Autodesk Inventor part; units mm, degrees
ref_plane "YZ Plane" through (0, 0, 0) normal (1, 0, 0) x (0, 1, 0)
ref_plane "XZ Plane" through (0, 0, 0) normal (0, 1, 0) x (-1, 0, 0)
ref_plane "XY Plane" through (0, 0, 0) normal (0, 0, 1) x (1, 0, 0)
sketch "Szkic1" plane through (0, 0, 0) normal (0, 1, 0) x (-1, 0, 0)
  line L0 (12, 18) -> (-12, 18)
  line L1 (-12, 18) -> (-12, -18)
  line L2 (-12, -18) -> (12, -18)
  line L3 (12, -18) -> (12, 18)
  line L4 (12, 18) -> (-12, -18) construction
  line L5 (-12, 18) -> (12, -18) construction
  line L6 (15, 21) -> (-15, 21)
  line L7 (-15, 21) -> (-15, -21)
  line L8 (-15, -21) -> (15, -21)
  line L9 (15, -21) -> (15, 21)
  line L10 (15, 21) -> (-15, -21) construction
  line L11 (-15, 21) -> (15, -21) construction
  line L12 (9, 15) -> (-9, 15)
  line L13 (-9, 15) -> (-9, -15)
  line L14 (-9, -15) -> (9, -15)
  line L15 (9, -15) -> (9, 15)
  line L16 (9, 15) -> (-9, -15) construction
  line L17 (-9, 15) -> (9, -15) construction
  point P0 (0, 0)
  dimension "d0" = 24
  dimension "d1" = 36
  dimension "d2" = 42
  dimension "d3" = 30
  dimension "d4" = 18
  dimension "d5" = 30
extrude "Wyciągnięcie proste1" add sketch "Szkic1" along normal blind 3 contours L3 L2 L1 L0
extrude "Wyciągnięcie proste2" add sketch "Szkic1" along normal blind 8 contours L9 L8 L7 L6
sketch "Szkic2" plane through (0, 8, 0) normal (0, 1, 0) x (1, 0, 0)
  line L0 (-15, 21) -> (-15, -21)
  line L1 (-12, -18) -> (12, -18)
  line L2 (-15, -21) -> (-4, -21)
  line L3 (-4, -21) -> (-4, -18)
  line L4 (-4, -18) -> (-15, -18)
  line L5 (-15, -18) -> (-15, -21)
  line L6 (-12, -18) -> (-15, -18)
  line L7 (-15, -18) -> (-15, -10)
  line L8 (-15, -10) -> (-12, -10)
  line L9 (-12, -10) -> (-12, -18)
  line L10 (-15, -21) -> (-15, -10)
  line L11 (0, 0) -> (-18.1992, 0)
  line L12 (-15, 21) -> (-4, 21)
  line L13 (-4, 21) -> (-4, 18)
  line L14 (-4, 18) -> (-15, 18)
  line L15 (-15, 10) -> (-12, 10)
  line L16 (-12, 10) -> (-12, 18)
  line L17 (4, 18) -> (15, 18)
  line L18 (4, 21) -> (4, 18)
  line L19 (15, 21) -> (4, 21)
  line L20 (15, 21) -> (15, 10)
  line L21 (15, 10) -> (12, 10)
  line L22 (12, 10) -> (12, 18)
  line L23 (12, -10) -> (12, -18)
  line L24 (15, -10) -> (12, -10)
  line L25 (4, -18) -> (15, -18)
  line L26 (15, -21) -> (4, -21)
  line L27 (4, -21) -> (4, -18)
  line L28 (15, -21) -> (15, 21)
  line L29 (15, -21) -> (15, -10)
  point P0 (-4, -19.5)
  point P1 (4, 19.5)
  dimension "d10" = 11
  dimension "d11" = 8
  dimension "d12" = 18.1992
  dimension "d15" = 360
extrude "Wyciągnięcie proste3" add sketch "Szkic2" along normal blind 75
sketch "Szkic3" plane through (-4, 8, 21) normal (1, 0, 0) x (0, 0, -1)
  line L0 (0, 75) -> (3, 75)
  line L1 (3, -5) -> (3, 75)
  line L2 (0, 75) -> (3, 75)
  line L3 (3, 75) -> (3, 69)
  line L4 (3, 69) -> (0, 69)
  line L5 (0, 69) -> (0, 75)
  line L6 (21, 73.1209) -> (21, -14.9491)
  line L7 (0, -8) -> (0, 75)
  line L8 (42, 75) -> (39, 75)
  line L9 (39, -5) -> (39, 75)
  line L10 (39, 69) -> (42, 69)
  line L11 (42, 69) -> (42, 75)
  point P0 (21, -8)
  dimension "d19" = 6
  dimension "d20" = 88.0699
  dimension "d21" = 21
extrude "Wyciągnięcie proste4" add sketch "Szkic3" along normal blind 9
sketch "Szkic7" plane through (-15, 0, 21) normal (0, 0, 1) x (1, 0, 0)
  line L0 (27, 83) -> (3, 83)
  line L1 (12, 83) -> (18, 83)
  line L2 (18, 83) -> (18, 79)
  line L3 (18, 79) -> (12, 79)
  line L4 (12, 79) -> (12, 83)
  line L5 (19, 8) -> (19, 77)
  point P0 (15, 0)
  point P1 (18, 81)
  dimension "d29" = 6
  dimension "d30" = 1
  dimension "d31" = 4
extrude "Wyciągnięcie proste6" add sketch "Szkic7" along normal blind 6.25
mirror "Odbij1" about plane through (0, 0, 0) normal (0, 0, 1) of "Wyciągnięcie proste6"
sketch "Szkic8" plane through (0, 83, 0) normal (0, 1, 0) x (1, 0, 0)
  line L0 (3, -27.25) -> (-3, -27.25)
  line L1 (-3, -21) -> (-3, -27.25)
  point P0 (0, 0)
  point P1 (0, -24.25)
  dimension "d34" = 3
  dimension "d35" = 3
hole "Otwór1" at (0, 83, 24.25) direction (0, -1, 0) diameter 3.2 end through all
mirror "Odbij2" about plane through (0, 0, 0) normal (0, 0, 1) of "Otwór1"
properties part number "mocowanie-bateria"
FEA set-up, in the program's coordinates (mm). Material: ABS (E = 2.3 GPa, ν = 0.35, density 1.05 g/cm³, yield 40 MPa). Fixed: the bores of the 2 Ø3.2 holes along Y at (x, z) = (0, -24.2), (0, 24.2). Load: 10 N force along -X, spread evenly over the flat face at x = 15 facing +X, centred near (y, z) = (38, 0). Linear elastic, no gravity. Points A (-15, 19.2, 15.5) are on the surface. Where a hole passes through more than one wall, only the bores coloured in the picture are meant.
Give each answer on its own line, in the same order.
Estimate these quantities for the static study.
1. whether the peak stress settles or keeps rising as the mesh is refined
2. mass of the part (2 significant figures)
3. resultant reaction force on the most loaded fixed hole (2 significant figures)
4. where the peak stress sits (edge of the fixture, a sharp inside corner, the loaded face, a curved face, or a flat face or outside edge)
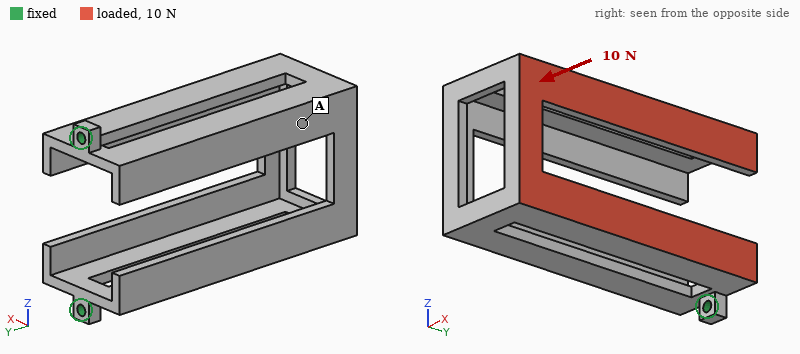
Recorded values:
keeps rising
23 g
5.0 N
edge of the fixture
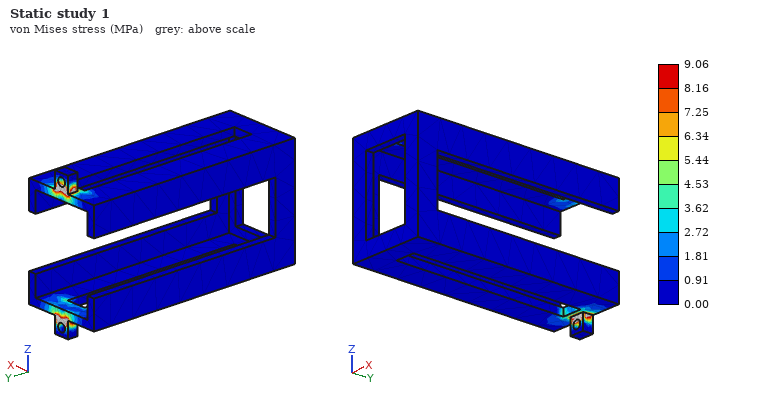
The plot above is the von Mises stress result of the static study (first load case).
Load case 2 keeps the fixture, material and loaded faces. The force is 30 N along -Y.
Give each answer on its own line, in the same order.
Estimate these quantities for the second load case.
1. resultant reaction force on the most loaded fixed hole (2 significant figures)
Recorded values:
15 N
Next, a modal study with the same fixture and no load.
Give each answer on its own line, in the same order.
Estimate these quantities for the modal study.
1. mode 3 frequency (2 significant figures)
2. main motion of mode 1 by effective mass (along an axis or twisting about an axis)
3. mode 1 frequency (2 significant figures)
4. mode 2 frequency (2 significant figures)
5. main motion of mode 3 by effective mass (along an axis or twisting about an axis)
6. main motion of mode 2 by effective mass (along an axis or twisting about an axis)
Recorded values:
340 Hz
along X
120 Hz
250 Hz
twisting about Y
along Z
